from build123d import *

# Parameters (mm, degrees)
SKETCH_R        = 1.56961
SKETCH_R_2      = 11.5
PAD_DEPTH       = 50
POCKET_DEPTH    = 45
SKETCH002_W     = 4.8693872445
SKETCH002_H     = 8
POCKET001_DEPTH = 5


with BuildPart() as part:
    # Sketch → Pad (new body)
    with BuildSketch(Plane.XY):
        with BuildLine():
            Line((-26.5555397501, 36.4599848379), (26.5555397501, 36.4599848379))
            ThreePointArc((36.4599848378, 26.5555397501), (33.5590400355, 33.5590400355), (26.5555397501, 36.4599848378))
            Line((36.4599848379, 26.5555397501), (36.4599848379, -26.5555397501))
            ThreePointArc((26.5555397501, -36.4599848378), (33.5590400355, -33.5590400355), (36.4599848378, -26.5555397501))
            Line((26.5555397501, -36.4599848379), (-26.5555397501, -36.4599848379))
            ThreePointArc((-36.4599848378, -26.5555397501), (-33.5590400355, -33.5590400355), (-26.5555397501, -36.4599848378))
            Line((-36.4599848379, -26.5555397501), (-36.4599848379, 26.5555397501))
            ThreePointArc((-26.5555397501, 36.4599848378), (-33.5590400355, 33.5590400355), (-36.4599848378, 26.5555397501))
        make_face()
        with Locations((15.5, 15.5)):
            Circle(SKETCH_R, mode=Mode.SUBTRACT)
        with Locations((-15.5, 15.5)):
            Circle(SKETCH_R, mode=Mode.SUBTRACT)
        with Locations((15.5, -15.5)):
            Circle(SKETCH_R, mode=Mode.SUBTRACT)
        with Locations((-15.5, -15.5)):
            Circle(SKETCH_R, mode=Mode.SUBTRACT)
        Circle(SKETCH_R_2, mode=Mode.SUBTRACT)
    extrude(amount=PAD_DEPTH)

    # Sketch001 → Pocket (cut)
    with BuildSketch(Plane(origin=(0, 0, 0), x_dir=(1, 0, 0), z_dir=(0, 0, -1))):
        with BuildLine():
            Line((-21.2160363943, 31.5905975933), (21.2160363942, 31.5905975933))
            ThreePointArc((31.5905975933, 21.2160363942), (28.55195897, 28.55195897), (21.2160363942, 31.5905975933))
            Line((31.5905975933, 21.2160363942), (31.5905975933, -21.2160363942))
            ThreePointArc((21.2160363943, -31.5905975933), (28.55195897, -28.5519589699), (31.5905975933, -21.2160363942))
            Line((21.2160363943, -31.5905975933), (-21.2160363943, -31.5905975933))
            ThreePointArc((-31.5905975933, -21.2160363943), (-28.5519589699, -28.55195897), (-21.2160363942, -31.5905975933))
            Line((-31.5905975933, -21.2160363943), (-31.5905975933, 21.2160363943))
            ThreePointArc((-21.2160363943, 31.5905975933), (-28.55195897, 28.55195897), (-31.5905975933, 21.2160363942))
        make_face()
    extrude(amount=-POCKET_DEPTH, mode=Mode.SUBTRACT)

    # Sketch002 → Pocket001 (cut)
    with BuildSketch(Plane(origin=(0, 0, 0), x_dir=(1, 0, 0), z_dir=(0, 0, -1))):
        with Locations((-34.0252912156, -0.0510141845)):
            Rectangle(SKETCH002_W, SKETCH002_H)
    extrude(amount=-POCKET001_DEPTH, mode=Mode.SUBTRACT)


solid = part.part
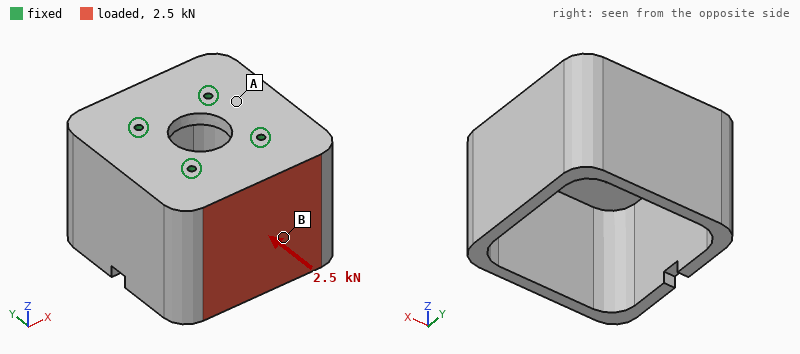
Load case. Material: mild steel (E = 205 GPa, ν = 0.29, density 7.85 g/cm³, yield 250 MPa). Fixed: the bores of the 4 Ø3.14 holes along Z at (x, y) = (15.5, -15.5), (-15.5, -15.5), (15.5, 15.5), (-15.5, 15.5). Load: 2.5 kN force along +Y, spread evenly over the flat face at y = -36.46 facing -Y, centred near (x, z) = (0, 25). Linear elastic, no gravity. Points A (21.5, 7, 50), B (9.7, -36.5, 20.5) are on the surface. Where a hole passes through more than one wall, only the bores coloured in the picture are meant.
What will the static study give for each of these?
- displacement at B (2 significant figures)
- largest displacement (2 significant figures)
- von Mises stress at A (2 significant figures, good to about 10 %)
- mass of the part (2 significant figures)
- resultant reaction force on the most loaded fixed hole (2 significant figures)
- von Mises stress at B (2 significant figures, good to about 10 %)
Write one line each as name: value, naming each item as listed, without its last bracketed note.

displacement at B: 34 µm
largest displacement: 56 µm
von Mises stress at A: 11 MPa
mass of the part: 660 g
resultant reaction force on the most loaded fixed hole: 1.2 kN
von Mises stress at B: 28 MPa
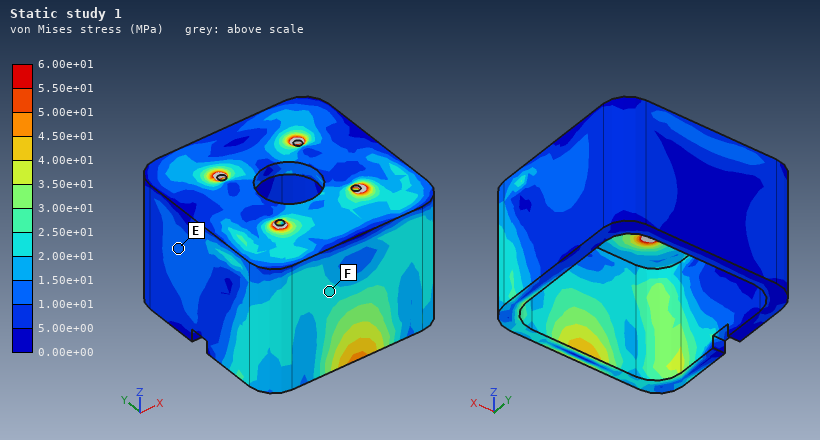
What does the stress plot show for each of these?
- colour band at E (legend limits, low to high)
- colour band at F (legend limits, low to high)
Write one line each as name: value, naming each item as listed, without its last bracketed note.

colour band at E: 1.00e+01 to 1.50e+01 MPa
colour band at F: 2.00e+01 to 2.50e+01 MPa
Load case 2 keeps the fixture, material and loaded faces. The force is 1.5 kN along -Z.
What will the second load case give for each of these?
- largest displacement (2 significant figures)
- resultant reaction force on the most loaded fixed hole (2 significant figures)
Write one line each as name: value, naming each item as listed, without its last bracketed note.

largest displacement: 25 µm
resultant reaction force on the most loaded fixed hole: 1.1 kN
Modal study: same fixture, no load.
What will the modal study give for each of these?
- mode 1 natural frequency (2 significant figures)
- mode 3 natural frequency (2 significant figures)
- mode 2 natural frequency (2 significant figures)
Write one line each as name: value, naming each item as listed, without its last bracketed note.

mode 1 natural frequency: 2300 Hz
mode 3 natural frequency: 2500 Hz
mode 2 natural frequency: 2300 Hz
